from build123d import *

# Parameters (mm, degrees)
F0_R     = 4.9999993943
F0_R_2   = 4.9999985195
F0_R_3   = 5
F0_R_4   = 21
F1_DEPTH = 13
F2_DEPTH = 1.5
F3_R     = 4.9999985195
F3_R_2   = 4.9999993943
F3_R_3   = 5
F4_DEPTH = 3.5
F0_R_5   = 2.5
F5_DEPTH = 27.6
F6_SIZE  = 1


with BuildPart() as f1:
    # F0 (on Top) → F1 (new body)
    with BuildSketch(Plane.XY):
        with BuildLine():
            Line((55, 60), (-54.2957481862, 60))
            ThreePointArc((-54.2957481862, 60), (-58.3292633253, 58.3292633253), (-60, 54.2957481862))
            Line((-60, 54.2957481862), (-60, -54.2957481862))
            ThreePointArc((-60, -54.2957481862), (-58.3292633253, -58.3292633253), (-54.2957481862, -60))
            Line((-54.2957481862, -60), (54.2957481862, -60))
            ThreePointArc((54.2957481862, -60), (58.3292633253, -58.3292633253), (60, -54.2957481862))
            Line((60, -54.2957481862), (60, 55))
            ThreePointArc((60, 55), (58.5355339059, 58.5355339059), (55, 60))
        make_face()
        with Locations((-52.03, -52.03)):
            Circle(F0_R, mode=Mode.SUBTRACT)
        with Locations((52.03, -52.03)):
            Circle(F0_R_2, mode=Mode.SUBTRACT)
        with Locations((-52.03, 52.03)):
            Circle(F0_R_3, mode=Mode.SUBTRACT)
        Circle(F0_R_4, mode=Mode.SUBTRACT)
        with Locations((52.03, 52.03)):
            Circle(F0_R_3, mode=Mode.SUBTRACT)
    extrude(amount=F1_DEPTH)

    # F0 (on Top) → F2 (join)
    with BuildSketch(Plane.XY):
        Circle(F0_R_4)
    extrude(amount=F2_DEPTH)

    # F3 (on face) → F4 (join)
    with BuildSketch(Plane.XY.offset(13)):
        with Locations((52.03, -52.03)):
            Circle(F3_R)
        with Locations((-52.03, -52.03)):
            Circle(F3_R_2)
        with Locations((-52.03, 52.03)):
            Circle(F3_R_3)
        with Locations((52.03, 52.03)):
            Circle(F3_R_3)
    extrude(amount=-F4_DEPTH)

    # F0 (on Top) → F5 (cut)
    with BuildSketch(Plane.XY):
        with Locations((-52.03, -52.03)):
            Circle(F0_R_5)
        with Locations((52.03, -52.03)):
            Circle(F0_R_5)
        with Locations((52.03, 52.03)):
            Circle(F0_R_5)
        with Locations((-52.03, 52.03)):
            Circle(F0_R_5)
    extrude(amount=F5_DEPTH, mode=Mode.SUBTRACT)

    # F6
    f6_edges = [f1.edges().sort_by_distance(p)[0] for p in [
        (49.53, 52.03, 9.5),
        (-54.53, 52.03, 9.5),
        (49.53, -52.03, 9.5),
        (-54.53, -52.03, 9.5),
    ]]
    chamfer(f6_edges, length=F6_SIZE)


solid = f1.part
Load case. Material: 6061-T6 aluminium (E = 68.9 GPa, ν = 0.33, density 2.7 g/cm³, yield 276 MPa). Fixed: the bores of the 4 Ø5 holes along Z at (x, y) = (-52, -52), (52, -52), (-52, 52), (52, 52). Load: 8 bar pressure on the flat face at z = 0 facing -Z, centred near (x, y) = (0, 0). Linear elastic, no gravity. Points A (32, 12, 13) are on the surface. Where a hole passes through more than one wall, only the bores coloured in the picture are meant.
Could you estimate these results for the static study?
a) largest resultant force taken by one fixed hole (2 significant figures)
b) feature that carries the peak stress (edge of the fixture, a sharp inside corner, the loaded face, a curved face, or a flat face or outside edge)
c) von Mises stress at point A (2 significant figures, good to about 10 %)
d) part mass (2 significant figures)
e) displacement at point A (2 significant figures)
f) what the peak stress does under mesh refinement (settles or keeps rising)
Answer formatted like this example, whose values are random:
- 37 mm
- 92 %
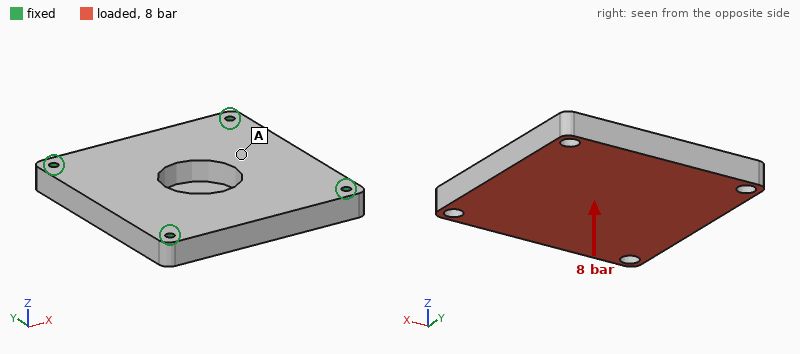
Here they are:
- 5.1 kN
- edge of the fixture
- 21 MPa
- 450 g
- 0.098 mm
- keeps rising
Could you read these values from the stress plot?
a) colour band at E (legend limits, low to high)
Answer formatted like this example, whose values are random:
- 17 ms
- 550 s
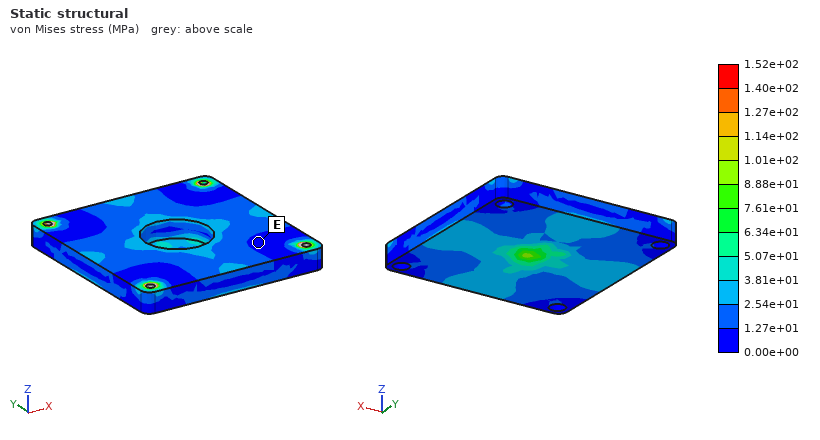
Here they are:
- 0.00e+00 to 1.27e+01 MPa
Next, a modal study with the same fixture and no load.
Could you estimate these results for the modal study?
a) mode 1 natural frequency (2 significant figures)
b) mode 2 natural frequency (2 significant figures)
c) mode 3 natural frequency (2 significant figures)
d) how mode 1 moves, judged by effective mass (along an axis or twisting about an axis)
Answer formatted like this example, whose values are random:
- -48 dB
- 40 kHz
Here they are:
- 2800 Hz
- 4500 Hz
- 4500 Hz
- along Z
